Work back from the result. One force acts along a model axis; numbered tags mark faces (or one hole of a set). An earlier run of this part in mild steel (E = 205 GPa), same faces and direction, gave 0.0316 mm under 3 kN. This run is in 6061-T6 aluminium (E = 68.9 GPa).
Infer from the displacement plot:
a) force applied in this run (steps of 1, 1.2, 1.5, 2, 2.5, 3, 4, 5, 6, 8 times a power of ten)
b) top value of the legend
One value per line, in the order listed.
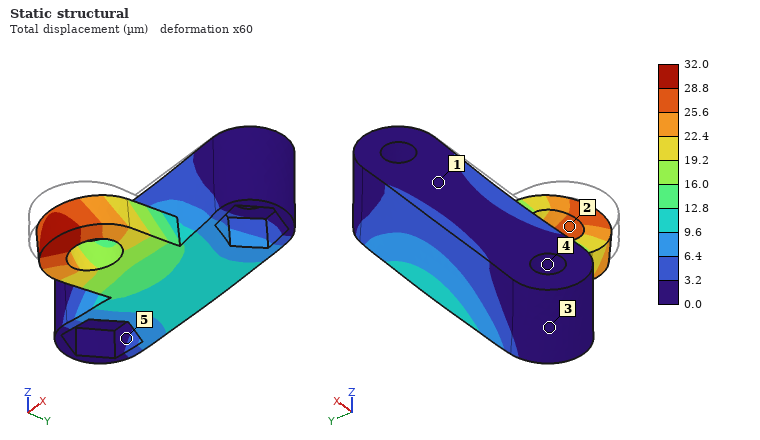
1 kN
32.0 µm
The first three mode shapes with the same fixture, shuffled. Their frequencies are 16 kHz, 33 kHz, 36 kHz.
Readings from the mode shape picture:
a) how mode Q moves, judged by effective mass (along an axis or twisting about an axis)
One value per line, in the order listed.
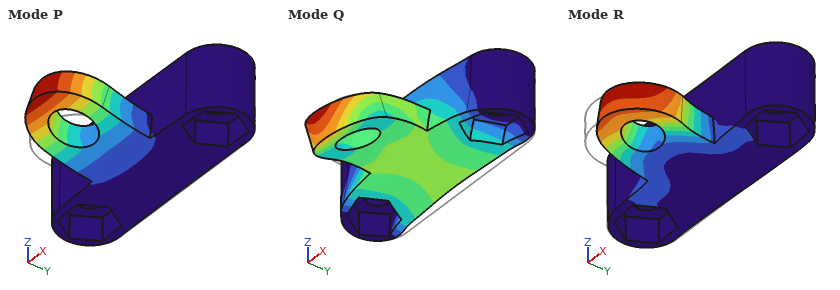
along Y
